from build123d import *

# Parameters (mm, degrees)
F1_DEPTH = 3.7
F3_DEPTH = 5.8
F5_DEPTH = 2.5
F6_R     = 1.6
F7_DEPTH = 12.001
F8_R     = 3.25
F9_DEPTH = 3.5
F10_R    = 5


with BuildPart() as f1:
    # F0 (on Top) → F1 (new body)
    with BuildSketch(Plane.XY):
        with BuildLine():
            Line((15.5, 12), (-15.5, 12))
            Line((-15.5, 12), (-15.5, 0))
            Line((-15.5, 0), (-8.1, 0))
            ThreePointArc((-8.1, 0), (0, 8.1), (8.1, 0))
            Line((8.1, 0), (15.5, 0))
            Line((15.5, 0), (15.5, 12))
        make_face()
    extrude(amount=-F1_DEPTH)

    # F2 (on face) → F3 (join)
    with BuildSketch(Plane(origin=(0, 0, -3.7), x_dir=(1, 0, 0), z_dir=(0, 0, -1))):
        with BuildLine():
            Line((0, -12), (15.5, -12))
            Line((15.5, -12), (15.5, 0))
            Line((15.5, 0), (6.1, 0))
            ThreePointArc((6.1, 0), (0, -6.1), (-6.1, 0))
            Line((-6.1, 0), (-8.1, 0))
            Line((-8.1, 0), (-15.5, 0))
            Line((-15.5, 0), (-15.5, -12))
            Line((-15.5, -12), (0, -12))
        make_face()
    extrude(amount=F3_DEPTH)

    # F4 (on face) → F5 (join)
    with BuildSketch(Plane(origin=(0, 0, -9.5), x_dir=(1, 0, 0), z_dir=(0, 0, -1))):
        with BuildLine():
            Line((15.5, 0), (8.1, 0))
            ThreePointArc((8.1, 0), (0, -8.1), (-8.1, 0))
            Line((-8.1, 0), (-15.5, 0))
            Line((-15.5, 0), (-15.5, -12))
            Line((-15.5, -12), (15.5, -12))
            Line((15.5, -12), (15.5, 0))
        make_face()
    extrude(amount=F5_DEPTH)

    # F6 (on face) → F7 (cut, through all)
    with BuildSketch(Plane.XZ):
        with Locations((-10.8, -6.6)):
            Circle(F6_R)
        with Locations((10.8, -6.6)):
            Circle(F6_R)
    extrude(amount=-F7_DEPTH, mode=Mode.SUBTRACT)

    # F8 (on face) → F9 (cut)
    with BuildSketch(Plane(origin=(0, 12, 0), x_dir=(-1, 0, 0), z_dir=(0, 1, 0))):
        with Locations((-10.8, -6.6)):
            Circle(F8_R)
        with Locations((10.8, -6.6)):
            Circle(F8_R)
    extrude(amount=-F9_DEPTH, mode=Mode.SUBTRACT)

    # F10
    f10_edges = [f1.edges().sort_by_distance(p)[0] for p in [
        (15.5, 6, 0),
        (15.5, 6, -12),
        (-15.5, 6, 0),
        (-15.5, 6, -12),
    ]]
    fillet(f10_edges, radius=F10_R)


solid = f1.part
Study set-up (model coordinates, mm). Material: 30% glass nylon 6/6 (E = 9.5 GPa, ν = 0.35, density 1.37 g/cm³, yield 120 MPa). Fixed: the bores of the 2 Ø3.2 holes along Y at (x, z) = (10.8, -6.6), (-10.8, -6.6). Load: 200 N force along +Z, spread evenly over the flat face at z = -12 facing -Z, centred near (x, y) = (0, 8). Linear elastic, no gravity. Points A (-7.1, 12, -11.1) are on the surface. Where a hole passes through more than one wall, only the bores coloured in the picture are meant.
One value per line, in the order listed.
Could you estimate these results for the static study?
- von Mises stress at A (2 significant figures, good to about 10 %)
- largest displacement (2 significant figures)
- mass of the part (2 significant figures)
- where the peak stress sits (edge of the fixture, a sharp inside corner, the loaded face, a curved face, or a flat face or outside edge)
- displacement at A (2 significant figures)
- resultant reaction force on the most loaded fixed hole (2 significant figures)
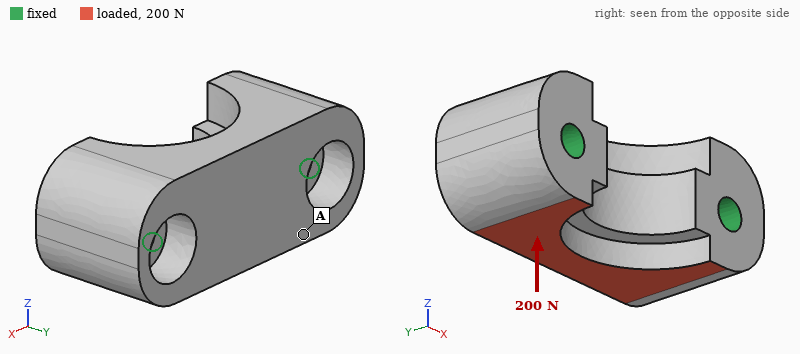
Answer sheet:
1.6 MPa
7.1 µm
3.9 g
edge of the fixture
5.5 µm
100 N
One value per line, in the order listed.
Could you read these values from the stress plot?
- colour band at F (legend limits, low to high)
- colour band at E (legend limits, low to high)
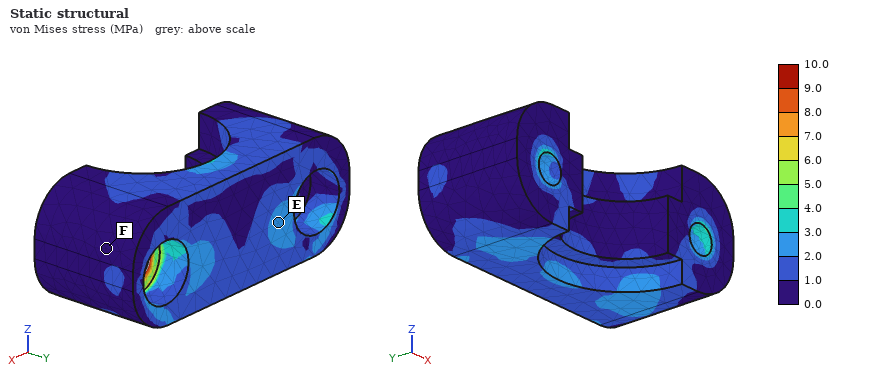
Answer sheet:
0.0 to 1.0 MPa
2.0 to 3.0 MPa
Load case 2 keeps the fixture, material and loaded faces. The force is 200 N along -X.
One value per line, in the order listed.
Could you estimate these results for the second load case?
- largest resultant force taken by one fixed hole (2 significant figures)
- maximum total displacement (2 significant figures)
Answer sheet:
110 N
3.6 µm
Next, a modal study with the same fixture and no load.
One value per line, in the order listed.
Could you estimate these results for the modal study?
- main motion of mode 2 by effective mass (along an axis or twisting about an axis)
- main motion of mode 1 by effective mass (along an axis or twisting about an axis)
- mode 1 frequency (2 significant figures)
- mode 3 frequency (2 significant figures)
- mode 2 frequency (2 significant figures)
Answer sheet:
along Y
along Z
21 kHz
35 kHz
31 kHz
